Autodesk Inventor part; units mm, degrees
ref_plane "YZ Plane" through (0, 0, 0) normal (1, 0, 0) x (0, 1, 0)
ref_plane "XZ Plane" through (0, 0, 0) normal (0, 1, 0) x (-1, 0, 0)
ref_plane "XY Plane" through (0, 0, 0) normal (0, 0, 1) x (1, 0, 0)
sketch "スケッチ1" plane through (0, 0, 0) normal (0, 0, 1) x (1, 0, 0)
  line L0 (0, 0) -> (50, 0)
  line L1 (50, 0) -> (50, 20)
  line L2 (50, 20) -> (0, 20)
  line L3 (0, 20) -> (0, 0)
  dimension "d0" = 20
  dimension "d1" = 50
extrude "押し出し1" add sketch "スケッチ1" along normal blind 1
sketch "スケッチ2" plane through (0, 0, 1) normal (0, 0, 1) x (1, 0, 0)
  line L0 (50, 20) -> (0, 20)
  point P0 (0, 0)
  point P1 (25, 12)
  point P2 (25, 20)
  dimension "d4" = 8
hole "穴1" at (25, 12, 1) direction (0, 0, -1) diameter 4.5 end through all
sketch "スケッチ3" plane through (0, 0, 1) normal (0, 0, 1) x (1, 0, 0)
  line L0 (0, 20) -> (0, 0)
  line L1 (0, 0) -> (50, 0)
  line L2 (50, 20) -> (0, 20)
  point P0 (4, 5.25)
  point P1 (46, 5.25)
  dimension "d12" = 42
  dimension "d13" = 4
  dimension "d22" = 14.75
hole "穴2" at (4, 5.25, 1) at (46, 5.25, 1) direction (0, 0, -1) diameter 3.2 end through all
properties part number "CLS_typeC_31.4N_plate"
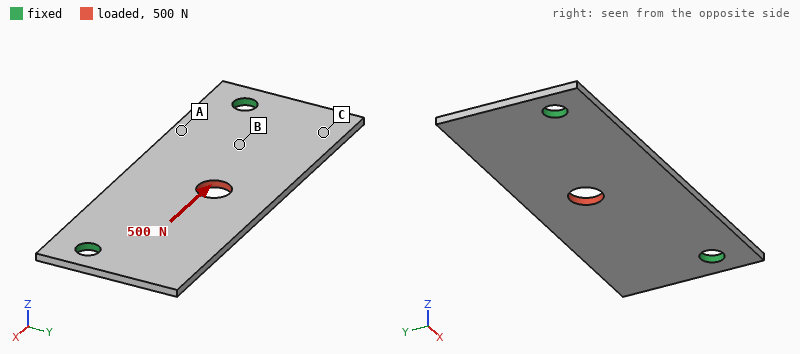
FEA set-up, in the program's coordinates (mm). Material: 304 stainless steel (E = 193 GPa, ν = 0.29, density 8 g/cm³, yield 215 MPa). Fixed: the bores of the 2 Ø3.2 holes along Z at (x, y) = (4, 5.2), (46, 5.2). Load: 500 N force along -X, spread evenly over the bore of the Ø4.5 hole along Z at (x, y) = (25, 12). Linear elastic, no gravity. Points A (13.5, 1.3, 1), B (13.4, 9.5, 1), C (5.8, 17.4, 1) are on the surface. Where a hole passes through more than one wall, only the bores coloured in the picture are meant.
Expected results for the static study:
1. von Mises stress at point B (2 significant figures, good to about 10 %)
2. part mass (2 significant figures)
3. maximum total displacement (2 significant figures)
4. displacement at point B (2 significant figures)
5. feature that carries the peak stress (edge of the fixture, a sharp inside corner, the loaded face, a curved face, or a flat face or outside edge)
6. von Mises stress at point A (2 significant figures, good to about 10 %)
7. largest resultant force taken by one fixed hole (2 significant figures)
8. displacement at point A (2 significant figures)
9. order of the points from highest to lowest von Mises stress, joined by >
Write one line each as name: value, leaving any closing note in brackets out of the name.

von Mises stress at point B: 22 MPa
part mass: 7.7 g
maximum total displacement: 3.1 µm
displacement at point B: 1.4 µm
feature that carries the peak stress: edge of the fixture
von Mises stress at point A: 13 MPa
largest resultant force taken by one fixed hole: 260 N
displacement at point A: 0.90 µm
order of the points from highest to lowest von Mises stress, joined by >: B > A > C
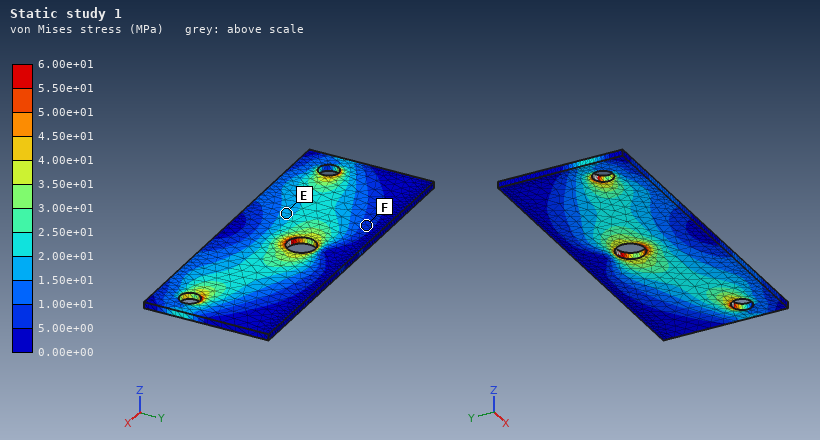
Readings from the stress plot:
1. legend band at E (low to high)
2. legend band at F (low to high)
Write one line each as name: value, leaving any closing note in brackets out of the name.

legend band at E: 1.50e+01 to 2.00e+01 MPa
legend band at F: 5.00e+00 to 1.00e+01 MPa
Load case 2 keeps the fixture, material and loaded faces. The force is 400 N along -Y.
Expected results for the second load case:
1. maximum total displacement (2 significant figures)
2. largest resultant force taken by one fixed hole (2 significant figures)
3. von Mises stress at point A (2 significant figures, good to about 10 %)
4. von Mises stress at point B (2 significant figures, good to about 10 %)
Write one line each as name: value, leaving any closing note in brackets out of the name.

maximum total displacement: 6.4 µm
largest resultant force taken by one fixed hole: 240 N
von Mises stress at point A: 9.0 MPa
von Mises stress at point B: 26 MPa
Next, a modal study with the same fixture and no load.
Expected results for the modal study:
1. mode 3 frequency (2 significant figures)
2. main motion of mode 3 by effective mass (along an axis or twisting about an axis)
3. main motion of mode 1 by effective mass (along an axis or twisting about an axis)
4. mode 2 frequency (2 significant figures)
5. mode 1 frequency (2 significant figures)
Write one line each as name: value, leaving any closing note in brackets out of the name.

mode 3 frequency: 4400 Hz
main motion of mode 3 by effective mass: twisting about Y
main motion of mode 1 by effective mass: along Z
mode 2 frequency: 3700 Hz
mode 1 frequency: 2200 Hz
